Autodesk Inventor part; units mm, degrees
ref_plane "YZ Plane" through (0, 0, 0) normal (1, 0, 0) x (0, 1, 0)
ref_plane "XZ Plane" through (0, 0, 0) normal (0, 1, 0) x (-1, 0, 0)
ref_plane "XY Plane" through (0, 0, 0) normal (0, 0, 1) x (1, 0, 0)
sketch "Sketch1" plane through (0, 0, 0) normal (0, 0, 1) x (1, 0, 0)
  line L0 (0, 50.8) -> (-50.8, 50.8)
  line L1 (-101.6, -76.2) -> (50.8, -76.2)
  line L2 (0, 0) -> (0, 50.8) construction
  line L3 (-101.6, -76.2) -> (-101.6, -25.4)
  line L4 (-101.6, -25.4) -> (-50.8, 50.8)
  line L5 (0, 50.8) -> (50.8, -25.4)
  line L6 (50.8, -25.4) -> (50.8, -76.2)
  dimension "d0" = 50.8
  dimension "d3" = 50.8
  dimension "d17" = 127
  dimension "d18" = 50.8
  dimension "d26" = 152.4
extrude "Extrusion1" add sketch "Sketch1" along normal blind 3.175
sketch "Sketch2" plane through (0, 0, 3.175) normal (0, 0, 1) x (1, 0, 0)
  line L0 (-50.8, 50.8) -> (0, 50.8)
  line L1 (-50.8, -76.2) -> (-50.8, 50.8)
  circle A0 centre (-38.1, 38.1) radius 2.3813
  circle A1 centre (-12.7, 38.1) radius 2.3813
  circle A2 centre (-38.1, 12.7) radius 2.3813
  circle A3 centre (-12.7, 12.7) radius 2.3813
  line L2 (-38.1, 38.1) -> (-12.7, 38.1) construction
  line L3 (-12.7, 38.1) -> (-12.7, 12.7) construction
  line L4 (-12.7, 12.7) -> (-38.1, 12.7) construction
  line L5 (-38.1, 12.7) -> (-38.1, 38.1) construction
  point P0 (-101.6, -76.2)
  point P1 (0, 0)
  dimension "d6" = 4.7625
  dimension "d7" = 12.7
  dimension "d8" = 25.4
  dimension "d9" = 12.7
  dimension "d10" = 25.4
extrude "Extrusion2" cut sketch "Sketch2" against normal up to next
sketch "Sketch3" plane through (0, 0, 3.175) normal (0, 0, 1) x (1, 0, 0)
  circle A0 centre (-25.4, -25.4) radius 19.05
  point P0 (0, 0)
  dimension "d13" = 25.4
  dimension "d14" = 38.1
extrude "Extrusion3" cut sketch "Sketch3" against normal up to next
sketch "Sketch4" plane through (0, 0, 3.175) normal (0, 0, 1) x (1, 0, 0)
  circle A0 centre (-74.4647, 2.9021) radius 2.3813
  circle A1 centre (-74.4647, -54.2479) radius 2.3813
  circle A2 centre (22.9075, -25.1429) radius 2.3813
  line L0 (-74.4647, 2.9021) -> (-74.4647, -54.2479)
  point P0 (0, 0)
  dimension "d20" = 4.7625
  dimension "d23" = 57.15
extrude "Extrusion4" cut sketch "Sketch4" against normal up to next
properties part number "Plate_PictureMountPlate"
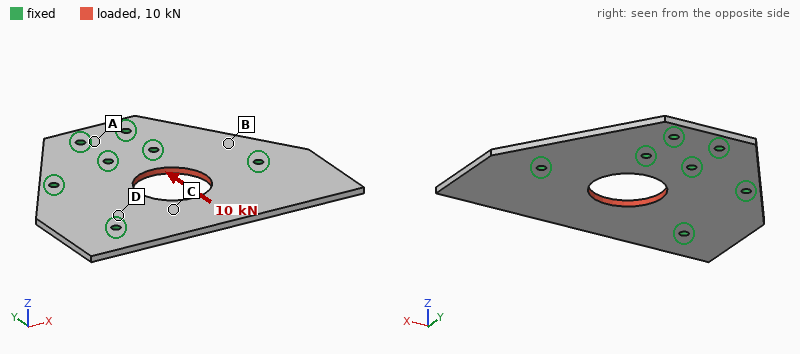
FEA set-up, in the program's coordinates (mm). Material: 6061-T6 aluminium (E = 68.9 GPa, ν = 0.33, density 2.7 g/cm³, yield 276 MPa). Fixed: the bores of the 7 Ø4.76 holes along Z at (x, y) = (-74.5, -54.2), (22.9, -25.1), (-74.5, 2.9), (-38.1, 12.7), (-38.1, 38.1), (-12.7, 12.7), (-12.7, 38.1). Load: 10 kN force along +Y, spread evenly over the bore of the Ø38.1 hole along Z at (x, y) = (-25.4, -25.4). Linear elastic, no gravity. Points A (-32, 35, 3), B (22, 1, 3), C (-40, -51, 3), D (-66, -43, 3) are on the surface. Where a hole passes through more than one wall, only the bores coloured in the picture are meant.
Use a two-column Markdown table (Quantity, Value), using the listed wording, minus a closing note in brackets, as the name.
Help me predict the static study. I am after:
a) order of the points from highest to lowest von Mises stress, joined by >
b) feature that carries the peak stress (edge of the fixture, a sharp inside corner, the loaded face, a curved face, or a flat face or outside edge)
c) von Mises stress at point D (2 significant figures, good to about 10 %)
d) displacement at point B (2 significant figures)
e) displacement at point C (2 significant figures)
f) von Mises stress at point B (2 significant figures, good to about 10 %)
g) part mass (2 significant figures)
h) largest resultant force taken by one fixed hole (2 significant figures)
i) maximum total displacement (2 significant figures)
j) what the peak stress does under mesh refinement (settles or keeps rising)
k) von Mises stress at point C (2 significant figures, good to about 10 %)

| Quantity | Value |
|---|---|
| order of the points from highest to lowest von Mises stress, joined by > | C > D > B > A |
| feature that carries the peak stress | edge of the fixture |
| von Mises stress at point D | 17 MPa |
| displacement at point B | 8.5 µm |
| displacement at point C | 27 µm |
| von Mises stress at point B | 9.3 MPa |
| part mass | 120 g |
| largest resultant force taken by one fixed hole | 2.4 kN |
| maximum total displacement | 37 µm |
| what the peak stress does under mesh refinement | keeps rising |
| von Mises stress at point C | 27 MPa |
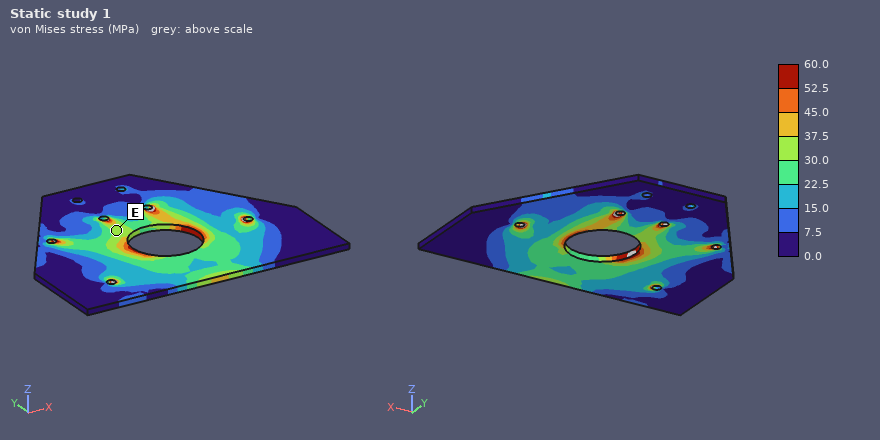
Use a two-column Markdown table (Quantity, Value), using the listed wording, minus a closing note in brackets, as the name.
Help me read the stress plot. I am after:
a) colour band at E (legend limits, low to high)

| Quantity | Value |
|---|---|
| colour band at E | 30.0 to 37.5 MPa |
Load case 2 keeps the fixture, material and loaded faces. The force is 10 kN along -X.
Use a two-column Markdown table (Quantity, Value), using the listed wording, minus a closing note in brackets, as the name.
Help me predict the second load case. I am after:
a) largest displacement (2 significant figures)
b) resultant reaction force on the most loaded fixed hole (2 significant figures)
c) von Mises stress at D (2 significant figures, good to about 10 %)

| Quantity | Value |
|---|---|
| largest displacement | 24 µm |
| resultant reaction force on the most loaded fixed hole | 3.0 kN |
| von Mises stress at D | 25 MPa |
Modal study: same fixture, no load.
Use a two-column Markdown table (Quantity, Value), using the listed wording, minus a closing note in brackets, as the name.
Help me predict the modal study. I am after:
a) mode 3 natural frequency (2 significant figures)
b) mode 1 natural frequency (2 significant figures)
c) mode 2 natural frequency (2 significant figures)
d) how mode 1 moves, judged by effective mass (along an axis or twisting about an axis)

| Quantity | Value |
|---|---|
| mode 3 natural frequency | 2900 Hz |
| mode 1 natural frequency | 950 Hz |
| mode 2 natural frequency | 1500 Hz |
| how mode 1 moves, judged by effective mass | along Z |
